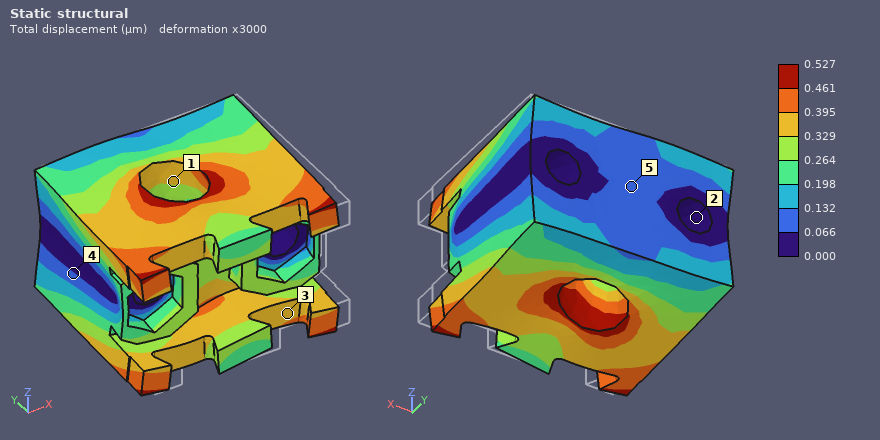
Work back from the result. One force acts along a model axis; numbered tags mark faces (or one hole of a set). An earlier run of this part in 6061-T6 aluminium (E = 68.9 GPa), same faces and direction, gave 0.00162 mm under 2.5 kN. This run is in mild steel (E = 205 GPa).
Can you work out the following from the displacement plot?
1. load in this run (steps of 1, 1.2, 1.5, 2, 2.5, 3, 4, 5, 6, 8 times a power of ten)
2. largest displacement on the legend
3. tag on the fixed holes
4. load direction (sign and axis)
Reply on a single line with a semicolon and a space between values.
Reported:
2.5 kN; 0.527 µm; 2; -X
